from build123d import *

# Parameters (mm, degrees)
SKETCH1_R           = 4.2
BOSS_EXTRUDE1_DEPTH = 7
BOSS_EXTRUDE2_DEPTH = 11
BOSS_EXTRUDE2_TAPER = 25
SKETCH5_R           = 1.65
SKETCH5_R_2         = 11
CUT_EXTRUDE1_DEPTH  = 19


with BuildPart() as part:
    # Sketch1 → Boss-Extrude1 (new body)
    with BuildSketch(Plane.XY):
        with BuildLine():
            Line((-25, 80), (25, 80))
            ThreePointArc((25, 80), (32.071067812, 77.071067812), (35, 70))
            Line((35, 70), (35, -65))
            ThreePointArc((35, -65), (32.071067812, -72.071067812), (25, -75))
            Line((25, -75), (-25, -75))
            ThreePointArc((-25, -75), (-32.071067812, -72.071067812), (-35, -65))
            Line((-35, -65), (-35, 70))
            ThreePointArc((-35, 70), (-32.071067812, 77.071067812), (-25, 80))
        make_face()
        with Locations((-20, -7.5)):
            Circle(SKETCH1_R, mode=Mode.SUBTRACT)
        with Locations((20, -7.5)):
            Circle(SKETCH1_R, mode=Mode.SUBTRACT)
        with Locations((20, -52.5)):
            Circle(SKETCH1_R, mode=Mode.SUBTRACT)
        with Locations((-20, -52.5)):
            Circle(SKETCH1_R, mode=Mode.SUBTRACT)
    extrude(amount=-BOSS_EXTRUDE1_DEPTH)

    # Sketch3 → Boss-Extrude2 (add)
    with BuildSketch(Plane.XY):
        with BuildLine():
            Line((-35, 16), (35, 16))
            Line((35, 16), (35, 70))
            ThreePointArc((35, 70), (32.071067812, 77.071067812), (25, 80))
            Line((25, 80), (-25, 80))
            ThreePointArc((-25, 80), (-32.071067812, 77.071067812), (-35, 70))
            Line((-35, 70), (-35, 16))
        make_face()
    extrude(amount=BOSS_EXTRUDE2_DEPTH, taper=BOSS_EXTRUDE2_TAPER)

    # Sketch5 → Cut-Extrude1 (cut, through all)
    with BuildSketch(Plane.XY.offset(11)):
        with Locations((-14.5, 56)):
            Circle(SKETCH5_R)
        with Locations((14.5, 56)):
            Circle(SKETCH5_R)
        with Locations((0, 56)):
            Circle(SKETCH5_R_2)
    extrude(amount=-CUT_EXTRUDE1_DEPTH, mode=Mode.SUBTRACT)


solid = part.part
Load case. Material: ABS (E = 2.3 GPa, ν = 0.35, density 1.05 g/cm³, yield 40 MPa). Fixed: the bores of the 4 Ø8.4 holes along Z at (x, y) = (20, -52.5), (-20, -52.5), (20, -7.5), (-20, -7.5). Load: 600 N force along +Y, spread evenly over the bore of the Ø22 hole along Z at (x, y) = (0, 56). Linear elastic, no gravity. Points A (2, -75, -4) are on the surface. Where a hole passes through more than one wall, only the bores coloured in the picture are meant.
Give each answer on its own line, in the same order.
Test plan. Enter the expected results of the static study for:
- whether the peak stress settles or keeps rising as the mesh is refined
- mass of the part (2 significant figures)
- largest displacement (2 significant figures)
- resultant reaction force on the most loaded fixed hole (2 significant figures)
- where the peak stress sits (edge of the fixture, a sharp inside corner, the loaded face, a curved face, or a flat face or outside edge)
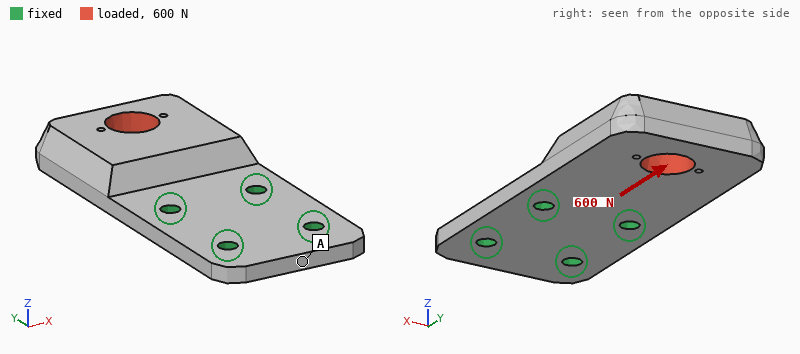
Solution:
keeps rising
110 g
1.2 mm
270 N
edge of the fixture
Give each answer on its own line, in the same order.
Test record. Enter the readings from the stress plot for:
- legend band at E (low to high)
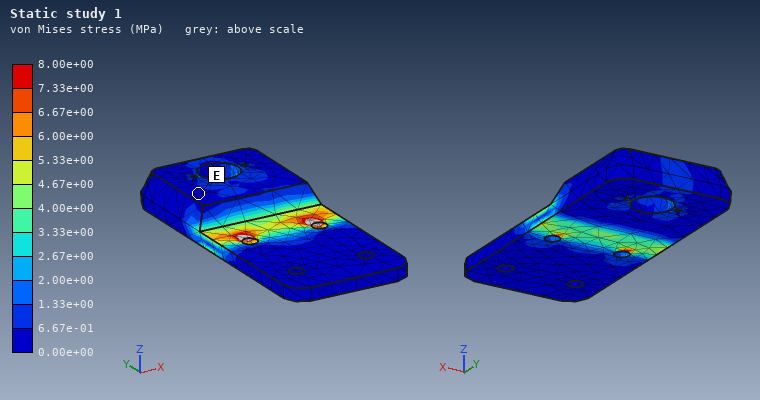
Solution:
0.00e+00 to 6.67e-01 MPa
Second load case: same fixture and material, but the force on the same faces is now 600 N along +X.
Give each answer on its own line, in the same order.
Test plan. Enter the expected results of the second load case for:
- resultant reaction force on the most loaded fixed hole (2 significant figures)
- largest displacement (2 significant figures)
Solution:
780 N
0.30 mm
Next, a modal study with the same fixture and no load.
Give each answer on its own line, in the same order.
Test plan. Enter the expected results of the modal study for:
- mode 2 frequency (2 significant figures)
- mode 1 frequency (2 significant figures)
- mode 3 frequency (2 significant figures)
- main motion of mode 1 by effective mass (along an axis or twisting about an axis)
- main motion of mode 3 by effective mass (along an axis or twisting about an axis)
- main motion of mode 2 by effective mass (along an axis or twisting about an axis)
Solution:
800 Hz
180 Hz
1100 Hz
along Z
along X
twisting about Y
